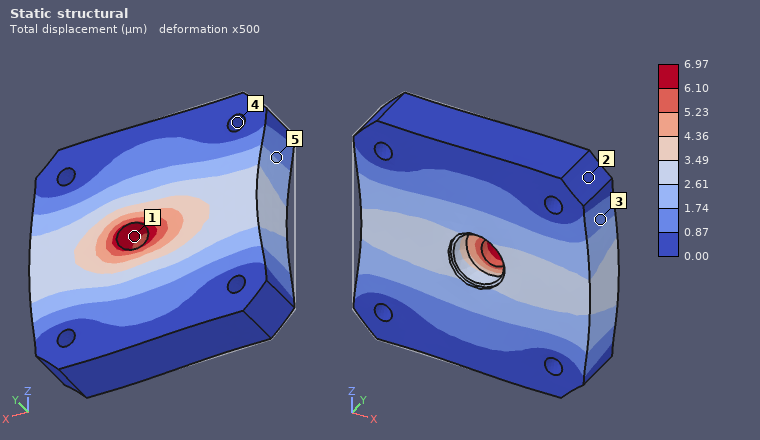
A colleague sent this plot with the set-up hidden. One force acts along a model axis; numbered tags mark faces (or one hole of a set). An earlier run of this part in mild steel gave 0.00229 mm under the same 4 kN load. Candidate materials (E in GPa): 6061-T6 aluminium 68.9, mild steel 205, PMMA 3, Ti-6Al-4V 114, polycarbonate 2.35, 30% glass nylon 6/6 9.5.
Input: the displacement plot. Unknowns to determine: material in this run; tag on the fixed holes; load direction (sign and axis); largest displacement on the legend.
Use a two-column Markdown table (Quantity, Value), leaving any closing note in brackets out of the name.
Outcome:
| Quantity | Value |
|---|---|
| material in this run | 6061-T6 aluminium |
| tag on the fixed holes | 4 |
| load direction | +X |
| largest displacement on the legend | 6.97 µm |
